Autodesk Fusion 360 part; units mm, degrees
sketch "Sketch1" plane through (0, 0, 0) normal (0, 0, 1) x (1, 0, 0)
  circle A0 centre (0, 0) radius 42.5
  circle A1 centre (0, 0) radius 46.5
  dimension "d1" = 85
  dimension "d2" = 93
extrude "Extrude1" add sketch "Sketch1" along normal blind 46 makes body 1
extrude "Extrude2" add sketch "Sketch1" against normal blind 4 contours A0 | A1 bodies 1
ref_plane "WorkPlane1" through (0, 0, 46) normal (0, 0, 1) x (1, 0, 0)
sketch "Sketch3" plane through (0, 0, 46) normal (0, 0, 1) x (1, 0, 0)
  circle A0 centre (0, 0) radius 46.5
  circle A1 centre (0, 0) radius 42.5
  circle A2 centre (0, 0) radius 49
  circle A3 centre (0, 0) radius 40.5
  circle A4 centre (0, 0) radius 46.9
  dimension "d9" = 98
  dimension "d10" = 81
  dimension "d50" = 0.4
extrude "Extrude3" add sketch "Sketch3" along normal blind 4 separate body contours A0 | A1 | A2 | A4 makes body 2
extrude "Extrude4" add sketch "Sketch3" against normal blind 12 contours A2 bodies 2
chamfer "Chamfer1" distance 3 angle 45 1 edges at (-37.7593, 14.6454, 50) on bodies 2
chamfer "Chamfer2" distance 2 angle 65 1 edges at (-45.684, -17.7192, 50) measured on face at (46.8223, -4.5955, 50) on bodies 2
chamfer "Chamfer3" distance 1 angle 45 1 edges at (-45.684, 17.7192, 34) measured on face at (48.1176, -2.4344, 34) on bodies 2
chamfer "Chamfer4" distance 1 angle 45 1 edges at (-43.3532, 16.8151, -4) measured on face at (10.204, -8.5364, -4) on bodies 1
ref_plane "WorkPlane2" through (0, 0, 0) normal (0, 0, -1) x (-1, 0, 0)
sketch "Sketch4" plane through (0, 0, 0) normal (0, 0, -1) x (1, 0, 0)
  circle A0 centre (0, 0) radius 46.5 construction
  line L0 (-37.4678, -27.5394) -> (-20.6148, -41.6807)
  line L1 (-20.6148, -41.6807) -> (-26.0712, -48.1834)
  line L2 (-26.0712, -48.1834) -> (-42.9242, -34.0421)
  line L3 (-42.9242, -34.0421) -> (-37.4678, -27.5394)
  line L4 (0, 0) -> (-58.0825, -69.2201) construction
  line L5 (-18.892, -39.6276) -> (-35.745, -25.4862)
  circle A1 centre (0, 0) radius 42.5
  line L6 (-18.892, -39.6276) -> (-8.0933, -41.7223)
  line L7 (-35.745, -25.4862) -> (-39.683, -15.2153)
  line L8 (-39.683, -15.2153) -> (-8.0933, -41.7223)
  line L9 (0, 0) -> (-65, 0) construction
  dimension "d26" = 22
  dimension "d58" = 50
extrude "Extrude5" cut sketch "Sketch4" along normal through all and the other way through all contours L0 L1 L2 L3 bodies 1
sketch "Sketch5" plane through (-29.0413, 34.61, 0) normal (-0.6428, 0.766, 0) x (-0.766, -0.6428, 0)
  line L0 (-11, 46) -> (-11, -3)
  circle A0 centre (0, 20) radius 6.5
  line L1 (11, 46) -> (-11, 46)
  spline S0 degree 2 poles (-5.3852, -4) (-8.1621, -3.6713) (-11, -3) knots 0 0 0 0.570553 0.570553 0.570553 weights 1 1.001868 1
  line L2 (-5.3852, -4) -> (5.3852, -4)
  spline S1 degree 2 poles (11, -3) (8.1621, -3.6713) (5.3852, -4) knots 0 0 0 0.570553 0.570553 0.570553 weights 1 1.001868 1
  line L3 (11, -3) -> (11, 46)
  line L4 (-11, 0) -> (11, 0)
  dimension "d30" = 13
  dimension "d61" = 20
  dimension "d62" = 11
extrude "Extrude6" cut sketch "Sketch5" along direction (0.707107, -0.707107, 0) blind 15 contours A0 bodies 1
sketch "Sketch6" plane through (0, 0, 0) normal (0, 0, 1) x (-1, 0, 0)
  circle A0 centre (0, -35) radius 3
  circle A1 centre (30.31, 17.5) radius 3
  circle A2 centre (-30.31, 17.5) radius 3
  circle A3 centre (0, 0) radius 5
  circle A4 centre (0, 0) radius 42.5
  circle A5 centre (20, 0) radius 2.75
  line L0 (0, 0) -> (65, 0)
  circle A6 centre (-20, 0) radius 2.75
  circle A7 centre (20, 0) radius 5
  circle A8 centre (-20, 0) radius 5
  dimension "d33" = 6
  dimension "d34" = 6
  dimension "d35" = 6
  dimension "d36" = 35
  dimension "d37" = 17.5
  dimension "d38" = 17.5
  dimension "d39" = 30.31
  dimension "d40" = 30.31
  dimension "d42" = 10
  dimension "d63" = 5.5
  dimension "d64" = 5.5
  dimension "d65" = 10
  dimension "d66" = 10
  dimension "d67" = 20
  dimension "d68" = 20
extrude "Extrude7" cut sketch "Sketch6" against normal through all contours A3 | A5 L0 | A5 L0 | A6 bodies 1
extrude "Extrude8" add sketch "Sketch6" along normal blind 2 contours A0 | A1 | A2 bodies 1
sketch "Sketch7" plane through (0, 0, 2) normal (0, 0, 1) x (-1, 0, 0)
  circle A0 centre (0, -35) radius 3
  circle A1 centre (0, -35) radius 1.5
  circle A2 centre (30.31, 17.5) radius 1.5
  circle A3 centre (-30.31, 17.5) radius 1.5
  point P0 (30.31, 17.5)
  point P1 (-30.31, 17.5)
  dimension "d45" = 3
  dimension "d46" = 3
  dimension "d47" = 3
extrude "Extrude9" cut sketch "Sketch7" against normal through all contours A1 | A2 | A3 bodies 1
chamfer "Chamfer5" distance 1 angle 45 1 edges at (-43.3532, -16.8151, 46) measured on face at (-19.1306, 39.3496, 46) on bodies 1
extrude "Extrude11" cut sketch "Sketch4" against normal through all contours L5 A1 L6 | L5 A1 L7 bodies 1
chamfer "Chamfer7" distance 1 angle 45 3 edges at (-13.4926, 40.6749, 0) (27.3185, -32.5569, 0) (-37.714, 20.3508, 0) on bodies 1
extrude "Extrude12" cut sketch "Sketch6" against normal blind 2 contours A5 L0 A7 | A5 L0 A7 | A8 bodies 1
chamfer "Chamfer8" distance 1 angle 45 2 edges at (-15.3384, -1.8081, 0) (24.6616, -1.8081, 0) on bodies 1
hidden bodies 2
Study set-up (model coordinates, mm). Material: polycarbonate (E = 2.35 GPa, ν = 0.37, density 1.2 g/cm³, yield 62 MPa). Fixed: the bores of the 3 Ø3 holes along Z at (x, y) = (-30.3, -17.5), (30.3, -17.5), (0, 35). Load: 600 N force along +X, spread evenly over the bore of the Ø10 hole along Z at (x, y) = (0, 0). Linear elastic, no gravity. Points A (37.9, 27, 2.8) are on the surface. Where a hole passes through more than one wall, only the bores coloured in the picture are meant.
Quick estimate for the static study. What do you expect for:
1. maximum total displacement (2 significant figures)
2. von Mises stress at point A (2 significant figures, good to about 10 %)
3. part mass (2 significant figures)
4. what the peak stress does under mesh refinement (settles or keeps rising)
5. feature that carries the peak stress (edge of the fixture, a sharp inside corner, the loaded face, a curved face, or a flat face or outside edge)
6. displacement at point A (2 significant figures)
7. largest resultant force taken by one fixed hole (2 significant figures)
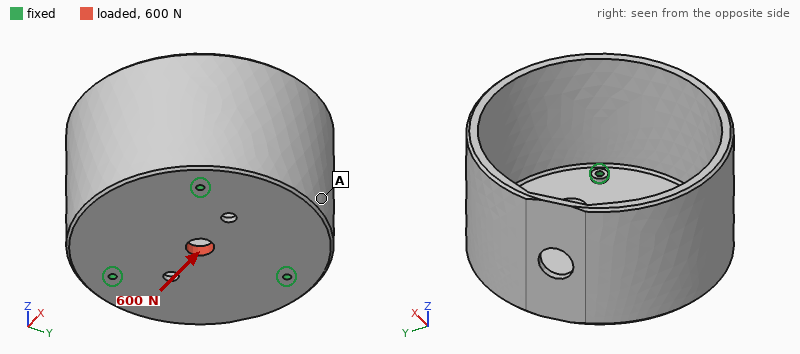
59 µm
0.66 MPa
91 g
keeps rising
edge of the fixture
19 µm
210 N
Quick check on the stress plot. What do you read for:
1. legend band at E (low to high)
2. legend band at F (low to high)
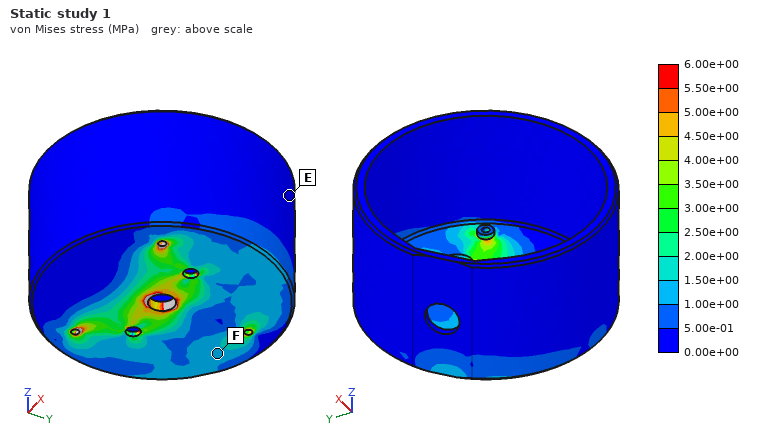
0.00e+00 to 5.00e-01 MPa
1.00e+00 to 1.50e+00 MPa
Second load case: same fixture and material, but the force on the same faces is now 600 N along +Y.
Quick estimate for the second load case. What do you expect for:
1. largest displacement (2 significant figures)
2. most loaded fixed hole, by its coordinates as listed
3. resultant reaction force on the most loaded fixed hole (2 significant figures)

57 µm
(0, 35)
230 N
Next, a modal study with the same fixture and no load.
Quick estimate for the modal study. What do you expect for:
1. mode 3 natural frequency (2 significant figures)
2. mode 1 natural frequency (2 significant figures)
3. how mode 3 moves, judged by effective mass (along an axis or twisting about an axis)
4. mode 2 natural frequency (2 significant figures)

950 Hz
470 Hz
along X
490 Hz
